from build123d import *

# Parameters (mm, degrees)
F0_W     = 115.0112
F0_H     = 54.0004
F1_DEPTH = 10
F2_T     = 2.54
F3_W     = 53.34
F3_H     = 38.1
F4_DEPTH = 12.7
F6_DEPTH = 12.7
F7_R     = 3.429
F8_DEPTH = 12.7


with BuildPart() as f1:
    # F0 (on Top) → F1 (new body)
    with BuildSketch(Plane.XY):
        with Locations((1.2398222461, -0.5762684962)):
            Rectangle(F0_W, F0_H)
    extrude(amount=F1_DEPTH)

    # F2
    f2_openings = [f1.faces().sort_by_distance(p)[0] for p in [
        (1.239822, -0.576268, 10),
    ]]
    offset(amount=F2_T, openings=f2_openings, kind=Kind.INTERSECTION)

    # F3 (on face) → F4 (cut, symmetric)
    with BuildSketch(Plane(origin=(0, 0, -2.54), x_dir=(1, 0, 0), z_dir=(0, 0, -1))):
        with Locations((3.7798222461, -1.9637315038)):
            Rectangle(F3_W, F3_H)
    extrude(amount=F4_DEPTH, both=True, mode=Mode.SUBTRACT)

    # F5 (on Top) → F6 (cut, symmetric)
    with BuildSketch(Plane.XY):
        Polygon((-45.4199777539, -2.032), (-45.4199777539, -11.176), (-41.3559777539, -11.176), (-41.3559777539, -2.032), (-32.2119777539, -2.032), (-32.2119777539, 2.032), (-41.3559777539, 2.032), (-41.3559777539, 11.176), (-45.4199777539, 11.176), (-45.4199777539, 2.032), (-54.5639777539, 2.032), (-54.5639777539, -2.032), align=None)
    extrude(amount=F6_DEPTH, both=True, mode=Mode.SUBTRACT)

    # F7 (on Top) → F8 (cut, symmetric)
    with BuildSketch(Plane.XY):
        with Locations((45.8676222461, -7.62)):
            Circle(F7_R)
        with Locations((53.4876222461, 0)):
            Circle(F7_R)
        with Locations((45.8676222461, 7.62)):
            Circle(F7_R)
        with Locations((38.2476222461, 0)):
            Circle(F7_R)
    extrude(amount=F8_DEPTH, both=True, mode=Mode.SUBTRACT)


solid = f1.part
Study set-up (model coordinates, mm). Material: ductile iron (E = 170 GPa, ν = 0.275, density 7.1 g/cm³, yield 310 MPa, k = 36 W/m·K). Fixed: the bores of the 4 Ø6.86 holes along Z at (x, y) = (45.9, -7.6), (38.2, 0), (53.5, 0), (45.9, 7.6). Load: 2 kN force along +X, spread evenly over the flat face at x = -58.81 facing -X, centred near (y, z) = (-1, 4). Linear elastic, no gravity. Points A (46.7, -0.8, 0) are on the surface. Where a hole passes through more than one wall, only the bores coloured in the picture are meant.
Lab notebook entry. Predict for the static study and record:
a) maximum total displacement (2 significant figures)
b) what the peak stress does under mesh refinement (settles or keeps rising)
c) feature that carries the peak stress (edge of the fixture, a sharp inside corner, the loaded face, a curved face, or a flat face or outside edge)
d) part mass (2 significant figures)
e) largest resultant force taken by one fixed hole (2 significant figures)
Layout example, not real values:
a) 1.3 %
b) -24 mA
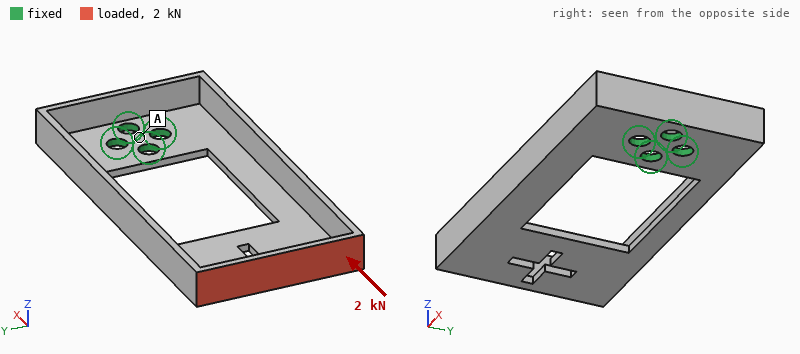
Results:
a) 0.48 mm
b) keeps rising
c) edge of the fixture
d) 150 g
e) 1.2 kN
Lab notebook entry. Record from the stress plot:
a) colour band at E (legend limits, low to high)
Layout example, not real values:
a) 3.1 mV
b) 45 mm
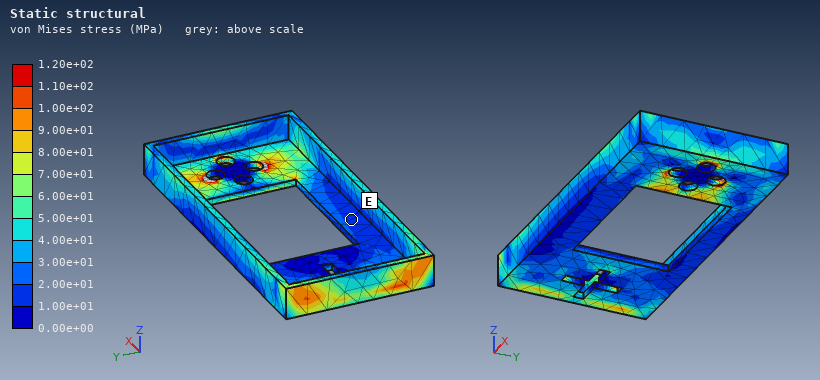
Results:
a) 1.00e+01 to 2.00e+01 MPa
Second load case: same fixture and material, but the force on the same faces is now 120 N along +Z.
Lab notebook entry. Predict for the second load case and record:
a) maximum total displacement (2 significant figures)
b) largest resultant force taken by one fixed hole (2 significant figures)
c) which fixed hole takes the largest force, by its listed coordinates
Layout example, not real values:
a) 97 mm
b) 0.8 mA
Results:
a) 0.63 mm
b) 640 N
c) (53.5, 0)
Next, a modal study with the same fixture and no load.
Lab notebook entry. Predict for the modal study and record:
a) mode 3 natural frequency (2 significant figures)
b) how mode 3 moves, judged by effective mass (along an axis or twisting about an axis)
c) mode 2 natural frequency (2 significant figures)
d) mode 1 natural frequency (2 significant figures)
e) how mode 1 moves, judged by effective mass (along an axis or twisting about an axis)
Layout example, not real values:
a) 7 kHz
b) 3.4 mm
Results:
a) 1100 Hz
b) along Y
c) 550 Hz
d) 320 Hz
e) along Z
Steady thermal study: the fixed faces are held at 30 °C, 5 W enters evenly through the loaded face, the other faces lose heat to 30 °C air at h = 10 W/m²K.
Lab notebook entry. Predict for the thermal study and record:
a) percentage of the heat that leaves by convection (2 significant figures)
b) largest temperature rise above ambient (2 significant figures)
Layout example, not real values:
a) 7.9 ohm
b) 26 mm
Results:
a) 75 %
b) 59 K
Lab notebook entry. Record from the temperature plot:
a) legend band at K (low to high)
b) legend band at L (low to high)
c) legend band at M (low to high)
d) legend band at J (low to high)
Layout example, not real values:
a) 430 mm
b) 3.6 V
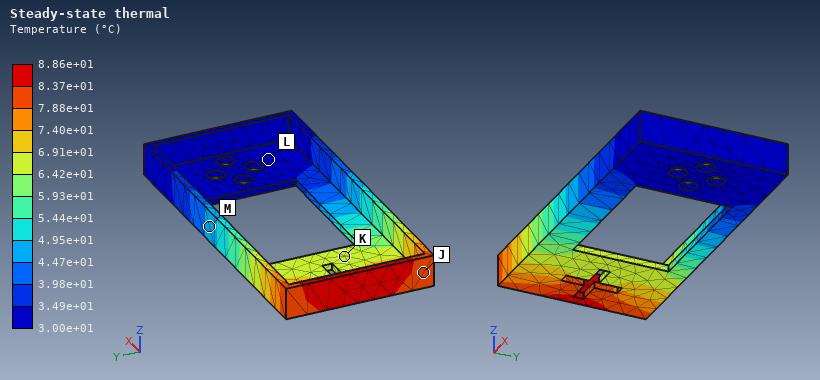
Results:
a) 6.42e+01 to 6.91e+01 °C
b) 3.00e+01 to 3.49e+01 °C
c) 4.47e+01 to 4.95e+01 °C
d) 7.88e+01 to 8.37e+01 °C
